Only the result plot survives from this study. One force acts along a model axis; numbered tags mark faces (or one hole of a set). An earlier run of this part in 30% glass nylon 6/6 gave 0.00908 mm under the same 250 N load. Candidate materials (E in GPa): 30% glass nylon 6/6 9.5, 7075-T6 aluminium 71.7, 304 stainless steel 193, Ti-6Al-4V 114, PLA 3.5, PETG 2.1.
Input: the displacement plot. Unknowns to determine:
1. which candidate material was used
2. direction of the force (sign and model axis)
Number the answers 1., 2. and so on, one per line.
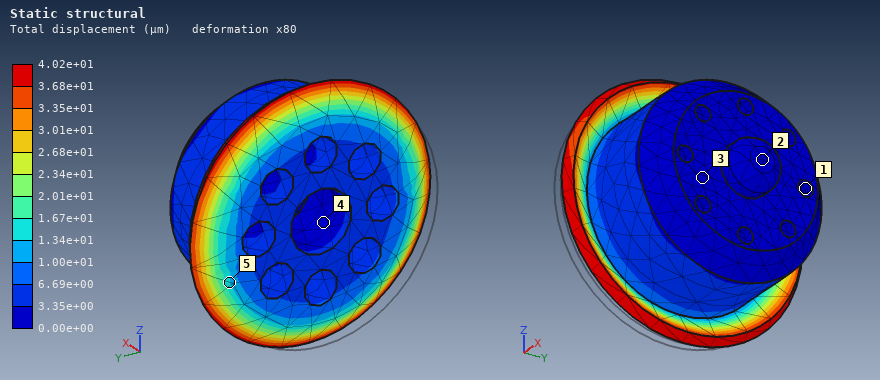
1. PETG
2. +X
